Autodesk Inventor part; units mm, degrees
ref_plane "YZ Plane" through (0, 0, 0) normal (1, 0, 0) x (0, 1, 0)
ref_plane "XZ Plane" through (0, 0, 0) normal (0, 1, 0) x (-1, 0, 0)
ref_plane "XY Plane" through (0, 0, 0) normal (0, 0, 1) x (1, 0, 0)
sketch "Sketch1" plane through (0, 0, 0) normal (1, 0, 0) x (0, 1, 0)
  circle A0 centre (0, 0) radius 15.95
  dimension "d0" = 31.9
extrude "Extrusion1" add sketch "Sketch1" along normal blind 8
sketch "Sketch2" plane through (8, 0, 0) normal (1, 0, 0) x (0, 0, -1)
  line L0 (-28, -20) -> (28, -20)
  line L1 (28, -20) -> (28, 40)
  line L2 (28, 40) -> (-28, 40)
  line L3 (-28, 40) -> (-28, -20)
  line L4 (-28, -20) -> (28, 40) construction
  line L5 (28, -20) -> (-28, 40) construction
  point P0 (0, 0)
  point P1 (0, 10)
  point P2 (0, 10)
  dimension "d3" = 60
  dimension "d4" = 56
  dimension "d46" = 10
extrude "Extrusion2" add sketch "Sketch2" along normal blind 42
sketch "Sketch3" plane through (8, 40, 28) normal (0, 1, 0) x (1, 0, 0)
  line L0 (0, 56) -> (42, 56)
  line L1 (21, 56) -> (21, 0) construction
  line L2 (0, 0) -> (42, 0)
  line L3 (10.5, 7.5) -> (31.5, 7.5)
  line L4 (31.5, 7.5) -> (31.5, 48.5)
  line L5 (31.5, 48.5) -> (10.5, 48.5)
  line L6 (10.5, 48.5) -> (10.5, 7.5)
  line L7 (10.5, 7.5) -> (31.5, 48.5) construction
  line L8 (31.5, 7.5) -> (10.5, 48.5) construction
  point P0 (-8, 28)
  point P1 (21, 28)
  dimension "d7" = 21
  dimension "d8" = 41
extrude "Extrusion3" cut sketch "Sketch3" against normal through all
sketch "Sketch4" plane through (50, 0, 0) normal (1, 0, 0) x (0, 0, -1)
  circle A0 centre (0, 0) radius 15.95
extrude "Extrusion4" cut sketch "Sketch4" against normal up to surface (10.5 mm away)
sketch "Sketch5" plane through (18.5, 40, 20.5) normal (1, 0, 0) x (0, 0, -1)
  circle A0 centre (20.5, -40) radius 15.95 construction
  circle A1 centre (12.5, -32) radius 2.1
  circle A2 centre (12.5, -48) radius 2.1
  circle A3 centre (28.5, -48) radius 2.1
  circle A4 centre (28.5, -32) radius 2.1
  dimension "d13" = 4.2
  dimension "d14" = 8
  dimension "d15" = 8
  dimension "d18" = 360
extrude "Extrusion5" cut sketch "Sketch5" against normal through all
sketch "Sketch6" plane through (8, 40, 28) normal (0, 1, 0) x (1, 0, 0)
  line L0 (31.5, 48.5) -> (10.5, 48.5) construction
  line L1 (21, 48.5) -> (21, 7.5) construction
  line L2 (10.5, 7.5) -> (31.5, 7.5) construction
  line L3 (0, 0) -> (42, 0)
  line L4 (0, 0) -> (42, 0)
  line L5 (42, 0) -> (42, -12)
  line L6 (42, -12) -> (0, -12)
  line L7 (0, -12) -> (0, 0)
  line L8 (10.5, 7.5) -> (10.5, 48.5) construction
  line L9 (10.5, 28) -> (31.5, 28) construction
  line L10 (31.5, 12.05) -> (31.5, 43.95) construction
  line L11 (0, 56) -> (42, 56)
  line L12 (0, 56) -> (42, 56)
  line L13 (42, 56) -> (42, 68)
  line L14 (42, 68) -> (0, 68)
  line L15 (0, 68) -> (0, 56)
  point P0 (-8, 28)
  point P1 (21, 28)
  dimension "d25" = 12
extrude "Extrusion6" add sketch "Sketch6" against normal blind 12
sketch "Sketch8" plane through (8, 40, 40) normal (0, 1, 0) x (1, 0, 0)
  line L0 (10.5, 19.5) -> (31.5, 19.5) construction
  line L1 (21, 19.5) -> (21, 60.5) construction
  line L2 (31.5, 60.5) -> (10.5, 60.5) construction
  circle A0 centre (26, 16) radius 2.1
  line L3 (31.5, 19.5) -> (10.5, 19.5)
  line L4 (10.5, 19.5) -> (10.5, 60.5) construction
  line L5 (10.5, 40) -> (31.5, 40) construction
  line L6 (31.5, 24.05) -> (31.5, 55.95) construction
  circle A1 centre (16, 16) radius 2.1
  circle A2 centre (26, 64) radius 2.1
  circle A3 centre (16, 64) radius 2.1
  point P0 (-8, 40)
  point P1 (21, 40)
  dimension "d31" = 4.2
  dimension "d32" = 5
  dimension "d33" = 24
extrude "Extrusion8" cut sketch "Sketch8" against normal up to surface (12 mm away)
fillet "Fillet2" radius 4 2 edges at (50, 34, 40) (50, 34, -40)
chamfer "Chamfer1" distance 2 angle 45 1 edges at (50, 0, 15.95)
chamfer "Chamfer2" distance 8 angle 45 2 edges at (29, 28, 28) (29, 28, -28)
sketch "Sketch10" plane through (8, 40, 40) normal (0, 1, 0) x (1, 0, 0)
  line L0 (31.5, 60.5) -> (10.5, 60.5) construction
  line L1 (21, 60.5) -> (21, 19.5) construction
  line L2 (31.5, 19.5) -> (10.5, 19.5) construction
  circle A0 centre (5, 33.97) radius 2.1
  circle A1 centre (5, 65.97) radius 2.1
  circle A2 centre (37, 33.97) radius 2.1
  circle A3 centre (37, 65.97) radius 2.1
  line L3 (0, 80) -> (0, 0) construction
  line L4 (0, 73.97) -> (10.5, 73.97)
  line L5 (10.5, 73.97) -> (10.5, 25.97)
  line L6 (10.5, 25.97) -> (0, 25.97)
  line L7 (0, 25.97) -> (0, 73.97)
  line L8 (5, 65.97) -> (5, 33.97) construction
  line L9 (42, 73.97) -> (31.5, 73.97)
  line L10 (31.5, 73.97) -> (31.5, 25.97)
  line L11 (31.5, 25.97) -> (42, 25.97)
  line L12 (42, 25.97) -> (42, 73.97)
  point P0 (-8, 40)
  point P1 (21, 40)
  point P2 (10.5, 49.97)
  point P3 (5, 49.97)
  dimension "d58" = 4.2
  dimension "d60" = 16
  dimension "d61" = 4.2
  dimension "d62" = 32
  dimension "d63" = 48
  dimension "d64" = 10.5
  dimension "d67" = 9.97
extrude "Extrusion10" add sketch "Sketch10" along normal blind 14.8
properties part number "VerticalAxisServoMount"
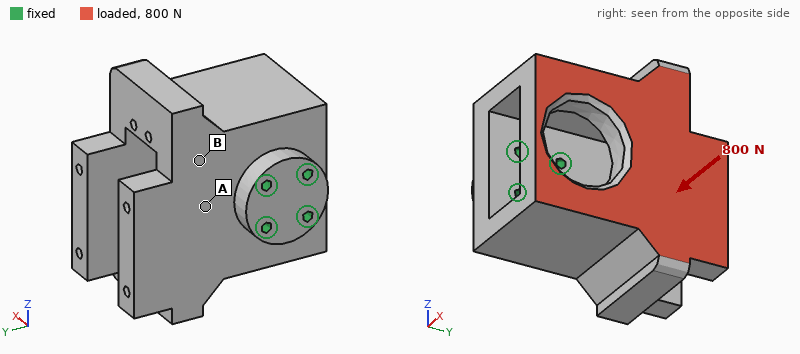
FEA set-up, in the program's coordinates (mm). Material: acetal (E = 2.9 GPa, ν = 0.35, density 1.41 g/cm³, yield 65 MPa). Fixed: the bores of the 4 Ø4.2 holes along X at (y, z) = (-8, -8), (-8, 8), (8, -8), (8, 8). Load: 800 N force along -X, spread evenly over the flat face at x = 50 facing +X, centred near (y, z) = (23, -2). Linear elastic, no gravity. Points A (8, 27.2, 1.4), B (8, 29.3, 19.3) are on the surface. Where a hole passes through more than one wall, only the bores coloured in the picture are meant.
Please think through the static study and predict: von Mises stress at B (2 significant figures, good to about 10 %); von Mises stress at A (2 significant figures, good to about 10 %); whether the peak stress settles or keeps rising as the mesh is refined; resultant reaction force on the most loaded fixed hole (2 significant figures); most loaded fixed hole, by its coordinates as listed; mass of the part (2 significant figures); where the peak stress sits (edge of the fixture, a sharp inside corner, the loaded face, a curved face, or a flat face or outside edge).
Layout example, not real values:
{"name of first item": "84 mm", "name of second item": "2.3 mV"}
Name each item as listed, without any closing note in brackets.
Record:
{"von Mises stress at B": "1.2 MPa", "von Mises stress at A": "3.0 MPa", "whether the peak stress settles or keeps rising as the mesh is refined": "keeps rising", "resultant reaction force on the most loaded fixed hole": "510 N", "most loaded fixed hole, by its coordinates as listed": "(8, -8)", "mass of the part": "160 g", "where the peak stress sits": "edge of the fixture"}
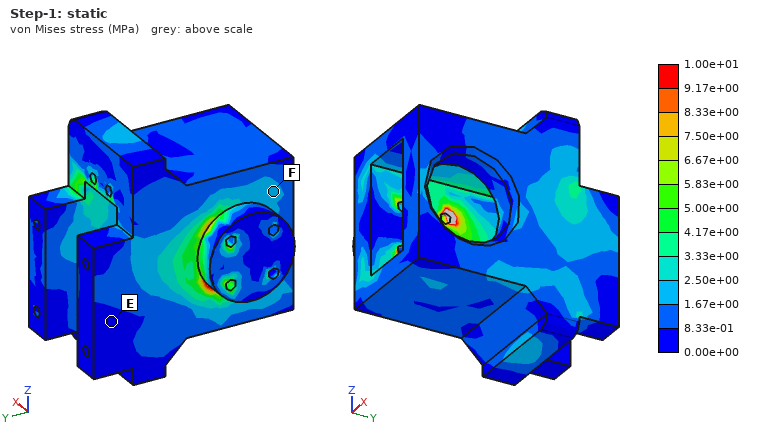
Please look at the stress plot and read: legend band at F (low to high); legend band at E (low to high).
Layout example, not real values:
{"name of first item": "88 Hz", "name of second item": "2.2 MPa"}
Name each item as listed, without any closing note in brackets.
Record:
{"legend band at F": "1.67e+00 to 2.50e+00 MPa", "legend band at E": "0.00e+00 to 8.33e-01 MPa"}
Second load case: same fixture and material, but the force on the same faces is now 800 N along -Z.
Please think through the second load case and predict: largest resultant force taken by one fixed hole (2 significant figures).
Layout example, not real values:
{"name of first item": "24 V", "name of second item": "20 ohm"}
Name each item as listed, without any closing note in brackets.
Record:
{"largest resultant force taken by one fixed hole": "710 N"}
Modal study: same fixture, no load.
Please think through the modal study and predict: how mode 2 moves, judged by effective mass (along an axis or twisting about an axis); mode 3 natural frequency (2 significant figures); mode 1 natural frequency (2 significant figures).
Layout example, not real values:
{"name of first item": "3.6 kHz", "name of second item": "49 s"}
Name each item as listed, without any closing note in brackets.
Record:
{"how mode 2 moves, judged by effective mass": "along Z", "mode 3 natural frequency": "1400 Hz", "mode 1 natural frequency": "800 Hz"}
